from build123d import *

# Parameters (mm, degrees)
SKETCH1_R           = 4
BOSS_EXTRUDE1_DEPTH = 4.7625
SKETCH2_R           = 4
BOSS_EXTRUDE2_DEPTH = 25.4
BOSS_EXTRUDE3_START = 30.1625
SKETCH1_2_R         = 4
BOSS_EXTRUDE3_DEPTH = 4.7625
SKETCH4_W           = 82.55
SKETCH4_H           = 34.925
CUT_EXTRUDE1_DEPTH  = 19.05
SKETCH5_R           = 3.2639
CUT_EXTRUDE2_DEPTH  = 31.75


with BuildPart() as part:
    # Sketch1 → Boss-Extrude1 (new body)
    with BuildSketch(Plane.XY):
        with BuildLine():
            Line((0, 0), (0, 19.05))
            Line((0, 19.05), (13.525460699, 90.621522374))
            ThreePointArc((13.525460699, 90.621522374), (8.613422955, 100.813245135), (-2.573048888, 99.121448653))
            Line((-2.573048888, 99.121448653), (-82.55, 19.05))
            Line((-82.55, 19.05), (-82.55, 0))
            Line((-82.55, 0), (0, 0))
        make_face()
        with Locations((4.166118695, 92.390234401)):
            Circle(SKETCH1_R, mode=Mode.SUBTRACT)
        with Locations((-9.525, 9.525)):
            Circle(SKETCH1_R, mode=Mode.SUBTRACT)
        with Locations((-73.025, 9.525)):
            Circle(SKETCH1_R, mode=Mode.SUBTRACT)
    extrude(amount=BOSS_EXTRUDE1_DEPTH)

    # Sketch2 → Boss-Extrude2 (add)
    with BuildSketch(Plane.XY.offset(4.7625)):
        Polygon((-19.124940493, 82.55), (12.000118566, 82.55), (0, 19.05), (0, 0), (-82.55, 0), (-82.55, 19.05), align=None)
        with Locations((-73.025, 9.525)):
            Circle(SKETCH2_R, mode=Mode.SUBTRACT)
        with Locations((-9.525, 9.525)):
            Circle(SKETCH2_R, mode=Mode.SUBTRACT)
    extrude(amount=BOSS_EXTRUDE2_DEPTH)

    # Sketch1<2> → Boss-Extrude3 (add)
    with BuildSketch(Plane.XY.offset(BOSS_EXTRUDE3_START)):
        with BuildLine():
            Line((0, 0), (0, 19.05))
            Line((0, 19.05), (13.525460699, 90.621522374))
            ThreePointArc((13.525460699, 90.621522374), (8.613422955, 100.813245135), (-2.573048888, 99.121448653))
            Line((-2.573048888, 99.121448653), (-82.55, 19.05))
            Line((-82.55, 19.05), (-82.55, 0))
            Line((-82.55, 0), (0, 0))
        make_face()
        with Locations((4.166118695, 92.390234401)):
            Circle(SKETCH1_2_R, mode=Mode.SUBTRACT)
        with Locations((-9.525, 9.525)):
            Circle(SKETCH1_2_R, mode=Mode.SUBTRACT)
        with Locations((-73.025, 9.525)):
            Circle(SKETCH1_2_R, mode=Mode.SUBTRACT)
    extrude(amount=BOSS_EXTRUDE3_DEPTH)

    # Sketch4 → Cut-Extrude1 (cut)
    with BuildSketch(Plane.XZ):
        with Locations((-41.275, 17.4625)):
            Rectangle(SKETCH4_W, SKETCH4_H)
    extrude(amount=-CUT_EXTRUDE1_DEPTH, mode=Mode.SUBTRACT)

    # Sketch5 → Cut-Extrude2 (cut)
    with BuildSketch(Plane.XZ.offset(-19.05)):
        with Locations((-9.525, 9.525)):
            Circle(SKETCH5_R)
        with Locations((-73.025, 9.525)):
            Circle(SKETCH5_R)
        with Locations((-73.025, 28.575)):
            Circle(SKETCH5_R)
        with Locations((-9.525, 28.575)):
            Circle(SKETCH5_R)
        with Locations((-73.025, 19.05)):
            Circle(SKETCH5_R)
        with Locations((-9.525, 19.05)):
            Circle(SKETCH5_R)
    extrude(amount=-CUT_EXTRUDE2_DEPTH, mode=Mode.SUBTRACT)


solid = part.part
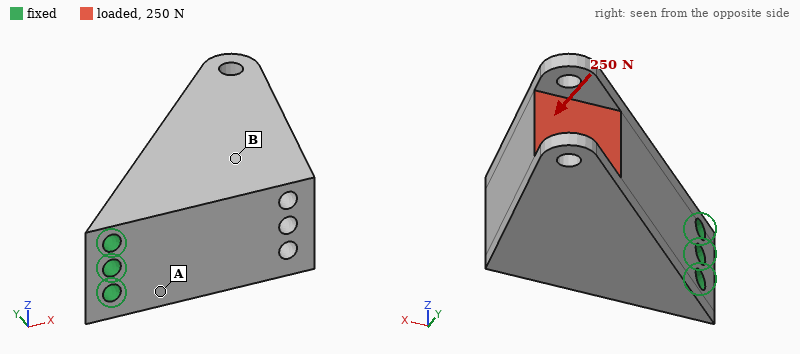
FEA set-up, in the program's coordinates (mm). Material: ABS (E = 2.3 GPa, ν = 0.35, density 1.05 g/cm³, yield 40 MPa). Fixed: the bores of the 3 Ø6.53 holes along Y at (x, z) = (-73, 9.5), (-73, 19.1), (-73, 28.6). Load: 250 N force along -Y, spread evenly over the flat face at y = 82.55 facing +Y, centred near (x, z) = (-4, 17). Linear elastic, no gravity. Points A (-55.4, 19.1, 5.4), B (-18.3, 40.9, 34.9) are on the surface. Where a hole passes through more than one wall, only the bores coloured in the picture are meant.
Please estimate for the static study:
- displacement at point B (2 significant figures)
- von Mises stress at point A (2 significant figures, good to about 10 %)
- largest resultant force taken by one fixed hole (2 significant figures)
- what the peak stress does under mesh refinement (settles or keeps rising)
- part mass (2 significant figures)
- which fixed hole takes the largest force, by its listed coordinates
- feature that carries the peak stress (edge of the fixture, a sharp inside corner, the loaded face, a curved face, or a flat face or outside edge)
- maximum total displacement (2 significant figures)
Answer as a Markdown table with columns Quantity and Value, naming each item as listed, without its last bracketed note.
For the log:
| Quantity | Value |
|---|---|
| displacement at point B | 0.58 mm |
| von Mises stress at point A | 4.8 MPa |
| largest resultant force taken by one fixed hole | 130 N |
| what the peak stress does under mesh refinement | keeps rising |
| part mass | 130 g |
| which fixed hole takes the largest force, by its listed coordinates | (-73, 19.1) |
| feature that carries the peak stress | edge of the fixture |
| maximum total displacement | 1.3 mm |
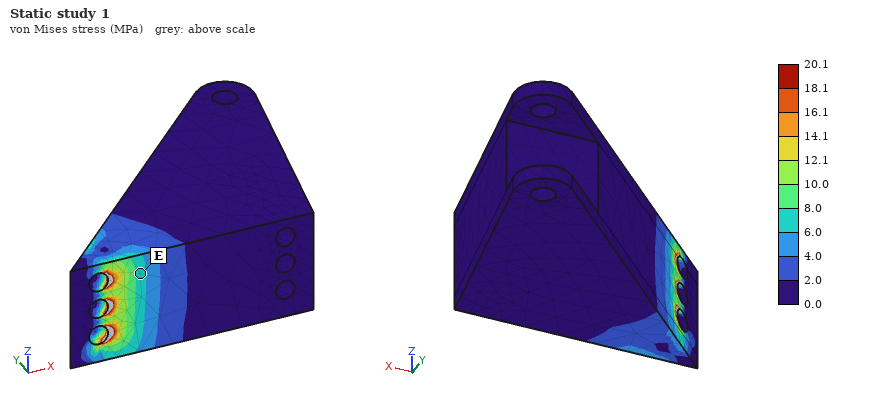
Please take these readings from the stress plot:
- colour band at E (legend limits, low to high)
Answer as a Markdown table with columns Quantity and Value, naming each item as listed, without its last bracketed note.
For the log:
| Quantity | Value |
|---|---|
| colour band at E | 6.0 to 8.0 MPa |
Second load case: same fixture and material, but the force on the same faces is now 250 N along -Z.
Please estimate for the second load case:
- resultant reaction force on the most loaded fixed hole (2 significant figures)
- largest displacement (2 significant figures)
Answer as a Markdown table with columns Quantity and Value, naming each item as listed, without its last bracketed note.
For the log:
| Quantity | Value |
|---|---|
| resultant reaction force on the most loaded fixed hole | 920 N |
| largest displacement | 0.68 mm |
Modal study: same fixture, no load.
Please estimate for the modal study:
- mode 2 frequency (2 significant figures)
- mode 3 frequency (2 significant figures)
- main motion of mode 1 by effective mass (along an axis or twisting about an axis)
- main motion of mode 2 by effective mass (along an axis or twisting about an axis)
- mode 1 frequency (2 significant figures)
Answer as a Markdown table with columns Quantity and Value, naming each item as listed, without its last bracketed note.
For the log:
| Quantity | Value |
|---|---|
| mode 2 frequency | 540 Hz |
| mode 3 frequency | 1100 Hz |
| main motion of mode 1 by effective mass | along Y |
| main motion of mode 2 by effective mass | along Z |
| mode 1 frequency | 290 Hz |
